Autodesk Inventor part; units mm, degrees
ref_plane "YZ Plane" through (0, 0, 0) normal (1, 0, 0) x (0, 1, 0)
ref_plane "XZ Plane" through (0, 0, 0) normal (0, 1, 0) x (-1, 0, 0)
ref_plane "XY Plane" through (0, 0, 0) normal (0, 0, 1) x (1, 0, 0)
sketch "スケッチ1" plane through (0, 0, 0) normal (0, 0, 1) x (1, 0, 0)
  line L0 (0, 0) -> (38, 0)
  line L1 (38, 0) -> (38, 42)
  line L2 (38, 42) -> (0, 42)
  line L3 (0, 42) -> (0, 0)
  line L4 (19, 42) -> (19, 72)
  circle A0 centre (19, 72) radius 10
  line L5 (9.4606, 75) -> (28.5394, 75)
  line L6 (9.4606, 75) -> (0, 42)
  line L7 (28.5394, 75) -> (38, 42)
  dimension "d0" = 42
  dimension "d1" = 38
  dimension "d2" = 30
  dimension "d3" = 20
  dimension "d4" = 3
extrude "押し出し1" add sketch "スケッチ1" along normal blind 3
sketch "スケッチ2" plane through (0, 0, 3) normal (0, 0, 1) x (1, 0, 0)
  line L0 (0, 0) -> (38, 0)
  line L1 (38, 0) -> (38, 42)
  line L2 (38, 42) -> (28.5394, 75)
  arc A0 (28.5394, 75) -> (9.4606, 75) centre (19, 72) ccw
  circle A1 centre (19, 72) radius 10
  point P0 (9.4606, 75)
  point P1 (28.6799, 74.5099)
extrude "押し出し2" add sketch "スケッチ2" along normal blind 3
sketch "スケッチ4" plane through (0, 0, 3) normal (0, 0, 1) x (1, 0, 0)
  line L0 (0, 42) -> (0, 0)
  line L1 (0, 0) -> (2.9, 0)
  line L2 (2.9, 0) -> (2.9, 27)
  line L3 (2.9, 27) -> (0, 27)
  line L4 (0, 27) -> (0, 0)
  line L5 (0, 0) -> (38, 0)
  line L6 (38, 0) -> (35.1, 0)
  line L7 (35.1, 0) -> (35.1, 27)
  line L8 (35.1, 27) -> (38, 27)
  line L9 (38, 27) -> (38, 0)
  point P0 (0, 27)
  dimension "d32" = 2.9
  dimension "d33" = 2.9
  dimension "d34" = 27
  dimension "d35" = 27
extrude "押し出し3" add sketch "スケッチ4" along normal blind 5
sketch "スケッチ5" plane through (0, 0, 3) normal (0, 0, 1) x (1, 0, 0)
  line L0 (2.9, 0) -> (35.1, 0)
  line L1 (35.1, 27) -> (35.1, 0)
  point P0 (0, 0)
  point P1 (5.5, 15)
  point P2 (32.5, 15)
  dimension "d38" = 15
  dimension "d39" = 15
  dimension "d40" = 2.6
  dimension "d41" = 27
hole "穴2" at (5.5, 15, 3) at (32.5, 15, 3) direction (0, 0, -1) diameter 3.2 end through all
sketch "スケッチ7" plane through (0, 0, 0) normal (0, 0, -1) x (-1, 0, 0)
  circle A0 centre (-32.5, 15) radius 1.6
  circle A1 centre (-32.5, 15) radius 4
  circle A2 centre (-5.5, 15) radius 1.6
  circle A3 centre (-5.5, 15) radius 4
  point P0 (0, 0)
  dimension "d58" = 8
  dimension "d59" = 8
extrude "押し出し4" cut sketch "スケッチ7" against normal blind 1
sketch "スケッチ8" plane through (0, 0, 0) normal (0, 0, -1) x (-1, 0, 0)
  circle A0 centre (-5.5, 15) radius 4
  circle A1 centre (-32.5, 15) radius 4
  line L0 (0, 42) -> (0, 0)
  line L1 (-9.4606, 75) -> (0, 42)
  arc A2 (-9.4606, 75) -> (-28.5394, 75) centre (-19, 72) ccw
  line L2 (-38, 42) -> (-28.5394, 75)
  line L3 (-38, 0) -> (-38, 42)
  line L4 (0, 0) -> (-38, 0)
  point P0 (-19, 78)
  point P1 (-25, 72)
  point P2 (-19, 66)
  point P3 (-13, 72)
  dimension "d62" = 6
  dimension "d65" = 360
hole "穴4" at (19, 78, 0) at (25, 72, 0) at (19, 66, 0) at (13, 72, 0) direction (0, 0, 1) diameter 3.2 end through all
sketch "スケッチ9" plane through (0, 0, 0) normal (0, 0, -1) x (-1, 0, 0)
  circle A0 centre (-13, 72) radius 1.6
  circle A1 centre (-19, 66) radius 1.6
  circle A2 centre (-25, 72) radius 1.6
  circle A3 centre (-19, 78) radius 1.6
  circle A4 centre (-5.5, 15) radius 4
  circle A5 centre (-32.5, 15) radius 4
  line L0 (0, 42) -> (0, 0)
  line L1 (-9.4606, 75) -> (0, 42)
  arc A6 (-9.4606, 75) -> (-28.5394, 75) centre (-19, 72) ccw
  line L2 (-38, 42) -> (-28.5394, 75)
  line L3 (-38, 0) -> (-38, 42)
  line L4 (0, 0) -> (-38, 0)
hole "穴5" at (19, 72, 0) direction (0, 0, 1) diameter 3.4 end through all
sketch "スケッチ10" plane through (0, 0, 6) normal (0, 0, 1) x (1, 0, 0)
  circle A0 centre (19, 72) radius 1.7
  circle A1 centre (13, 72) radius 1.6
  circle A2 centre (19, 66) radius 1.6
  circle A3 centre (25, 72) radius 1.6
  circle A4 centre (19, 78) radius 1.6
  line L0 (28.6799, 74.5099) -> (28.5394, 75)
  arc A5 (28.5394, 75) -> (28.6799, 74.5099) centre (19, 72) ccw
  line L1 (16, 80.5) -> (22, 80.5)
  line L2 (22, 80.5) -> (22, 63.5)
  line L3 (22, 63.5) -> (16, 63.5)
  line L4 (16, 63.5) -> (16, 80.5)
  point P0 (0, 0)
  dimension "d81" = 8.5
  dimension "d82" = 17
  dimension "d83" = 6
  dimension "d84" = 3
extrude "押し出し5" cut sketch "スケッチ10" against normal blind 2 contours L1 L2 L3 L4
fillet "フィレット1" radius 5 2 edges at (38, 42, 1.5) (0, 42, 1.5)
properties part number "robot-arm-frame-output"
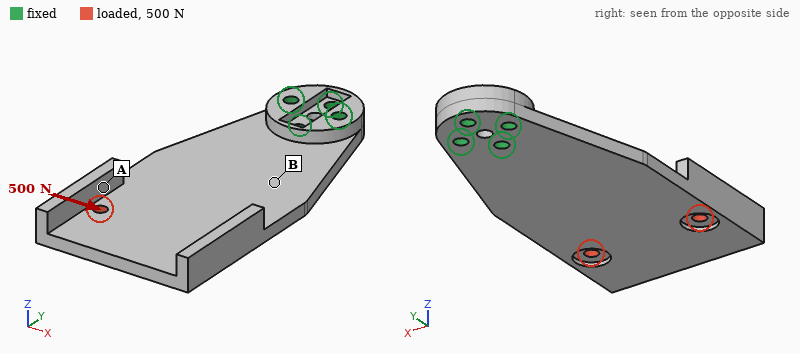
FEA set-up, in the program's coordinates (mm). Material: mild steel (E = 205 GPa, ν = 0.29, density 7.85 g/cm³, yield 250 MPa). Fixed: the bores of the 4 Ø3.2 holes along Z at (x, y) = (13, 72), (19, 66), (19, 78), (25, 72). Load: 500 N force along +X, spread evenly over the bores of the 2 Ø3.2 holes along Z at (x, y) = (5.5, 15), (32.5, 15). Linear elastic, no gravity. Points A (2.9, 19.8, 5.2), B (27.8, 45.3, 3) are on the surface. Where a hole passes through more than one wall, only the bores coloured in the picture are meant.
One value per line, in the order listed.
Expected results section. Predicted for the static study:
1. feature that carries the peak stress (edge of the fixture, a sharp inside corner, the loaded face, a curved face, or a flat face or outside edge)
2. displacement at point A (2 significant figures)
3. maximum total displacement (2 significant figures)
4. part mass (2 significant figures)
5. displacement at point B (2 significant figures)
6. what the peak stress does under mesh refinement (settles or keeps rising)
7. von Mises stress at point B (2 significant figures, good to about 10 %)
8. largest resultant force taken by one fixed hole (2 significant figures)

edge of the fixture
36 µm
52 µm
71 g
14 µm
keeps rising
21 MPa
1.4 kN
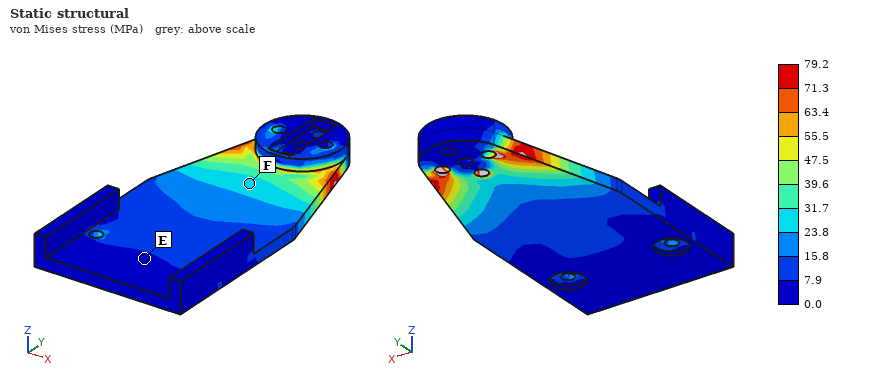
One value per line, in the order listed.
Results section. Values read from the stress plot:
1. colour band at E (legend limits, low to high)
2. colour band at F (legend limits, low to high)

0.0 to 7.9 MPa
23.8 to 31.7 MPa
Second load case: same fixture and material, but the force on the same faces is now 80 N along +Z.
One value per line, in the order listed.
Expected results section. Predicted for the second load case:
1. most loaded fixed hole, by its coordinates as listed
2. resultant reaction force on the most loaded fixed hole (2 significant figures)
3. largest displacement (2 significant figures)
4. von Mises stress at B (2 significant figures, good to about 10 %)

(19, 66)
340 N
0.33 mm
43 MPa
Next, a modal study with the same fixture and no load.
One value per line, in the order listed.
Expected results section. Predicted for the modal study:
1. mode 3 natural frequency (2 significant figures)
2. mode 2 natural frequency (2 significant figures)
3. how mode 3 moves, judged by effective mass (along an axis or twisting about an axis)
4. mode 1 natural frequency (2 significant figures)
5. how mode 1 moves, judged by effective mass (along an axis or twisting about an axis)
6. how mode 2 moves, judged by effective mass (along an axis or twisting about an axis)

3000 Hz
1600 Hz
along X
490 Hz
along Z
twisting about Y
